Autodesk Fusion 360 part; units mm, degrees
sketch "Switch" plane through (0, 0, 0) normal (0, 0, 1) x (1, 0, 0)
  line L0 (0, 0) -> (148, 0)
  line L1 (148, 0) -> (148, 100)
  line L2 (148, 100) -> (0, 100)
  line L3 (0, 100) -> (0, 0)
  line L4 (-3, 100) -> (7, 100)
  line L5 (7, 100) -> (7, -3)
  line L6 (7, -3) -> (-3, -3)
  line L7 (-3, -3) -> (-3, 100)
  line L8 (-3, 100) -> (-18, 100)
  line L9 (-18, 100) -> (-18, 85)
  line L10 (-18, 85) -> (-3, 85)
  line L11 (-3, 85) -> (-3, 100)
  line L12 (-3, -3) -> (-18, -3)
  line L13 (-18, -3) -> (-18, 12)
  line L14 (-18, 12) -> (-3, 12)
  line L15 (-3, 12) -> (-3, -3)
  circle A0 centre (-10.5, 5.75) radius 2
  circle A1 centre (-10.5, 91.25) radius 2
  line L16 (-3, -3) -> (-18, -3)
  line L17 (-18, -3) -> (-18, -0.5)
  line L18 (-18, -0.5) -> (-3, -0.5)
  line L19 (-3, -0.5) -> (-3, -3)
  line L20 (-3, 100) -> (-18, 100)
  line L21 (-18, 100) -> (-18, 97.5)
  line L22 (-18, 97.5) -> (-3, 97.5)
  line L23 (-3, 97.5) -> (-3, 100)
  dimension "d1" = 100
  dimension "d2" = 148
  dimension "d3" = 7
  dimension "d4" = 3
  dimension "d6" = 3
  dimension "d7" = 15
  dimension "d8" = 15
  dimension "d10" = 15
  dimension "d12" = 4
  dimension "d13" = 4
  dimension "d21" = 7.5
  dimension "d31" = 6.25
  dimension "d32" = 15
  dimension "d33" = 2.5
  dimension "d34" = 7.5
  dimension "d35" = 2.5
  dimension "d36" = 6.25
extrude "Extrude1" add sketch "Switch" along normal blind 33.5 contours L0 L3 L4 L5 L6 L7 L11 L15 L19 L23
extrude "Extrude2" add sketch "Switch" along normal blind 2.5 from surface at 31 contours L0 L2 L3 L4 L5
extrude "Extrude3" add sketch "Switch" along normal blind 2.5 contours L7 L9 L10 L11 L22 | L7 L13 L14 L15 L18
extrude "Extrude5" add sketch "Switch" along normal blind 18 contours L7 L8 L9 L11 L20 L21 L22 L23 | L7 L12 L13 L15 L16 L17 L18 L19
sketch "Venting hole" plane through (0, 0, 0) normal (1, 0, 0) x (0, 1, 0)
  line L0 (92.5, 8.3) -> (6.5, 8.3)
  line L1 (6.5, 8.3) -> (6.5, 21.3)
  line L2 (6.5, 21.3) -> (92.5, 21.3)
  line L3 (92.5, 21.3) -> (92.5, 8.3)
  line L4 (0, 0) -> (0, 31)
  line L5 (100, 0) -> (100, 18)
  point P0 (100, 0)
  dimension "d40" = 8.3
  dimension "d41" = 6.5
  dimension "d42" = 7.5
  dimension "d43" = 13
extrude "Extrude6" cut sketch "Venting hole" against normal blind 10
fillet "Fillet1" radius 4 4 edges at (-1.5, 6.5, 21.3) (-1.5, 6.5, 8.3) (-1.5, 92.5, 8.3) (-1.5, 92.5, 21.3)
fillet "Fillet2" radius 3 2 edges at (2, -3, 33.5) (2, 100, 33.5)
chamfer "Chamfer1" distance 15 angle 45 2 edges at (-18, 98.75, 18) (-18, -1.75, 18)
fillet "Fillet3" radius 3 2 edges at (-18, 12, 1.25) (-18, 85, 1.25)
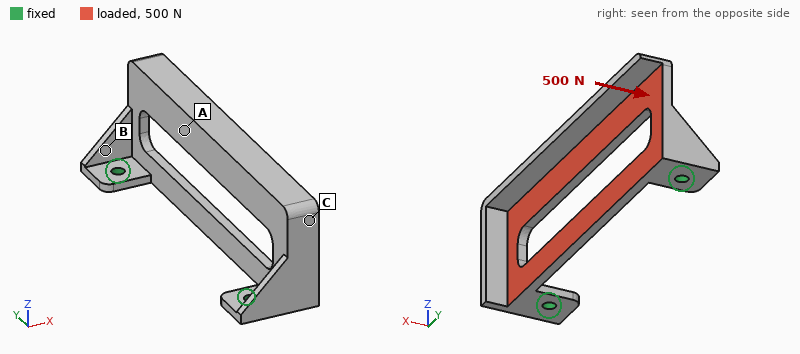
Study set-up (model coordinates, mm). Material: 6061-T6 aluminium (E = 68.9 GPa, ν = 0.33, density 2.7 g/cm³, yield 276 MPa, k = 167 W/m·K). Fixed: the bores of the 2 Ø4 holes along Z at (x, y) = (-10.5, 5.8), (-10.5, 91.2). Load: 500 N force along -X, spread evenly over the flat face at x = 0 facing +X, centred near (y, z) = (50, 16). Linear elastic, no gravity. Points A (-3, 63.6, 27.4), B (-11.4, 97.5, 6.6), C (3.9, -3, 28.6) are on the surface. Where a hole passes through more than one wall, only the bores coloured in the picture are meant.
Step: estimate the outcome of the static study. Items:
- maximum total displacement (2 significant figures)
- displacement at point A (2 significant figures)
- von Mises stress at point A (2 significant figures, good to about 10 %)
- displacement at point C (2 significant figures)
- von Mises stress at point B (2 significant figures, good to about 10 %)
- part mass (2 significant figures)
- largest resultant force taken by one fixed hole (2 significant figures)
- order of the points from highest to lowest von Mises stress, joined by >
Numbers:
0.42 mm
0.35 mm
25 MPa
0.21 mm
53 MPa
30 g
270 N
B > A > C
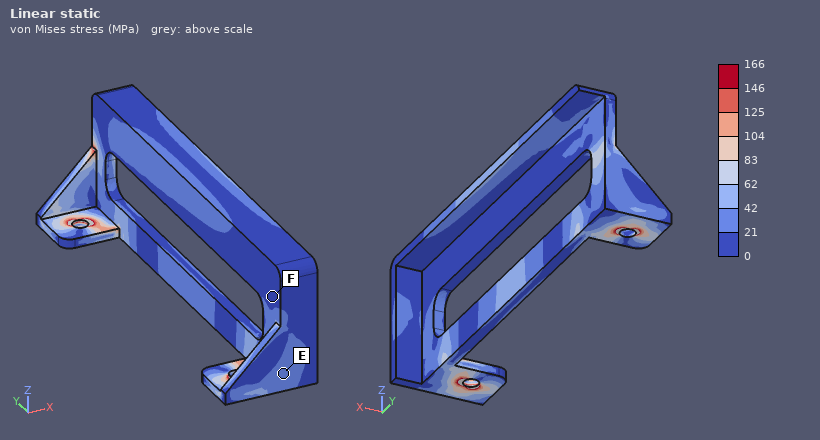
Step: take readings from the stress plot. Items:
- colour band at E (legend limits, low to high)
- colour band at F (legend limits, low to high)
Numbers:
21 to 42 MPa
0 to 21 MPa
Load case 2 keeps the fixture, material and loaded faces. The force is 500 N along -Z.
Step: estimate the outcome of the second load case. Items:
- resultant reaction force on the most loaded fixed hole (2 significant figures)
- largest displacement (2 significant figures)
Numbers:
260 N
0.19 mm
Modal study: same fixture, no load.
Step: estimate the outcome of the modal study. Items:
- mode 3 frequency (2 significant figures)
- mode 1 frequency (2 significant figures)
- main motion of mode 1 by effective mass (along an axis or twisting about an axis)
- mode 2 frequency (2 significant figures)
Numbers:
2400 Hz
1100 Hz
along X
2100 Hz
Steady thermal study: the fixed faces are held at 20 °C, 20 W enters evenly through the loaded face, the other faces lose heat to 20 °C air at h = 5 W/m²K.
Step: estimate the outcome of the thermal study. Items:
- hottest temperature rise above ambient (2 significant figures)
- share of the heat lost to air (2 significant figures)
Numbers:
37 K
4.2 %
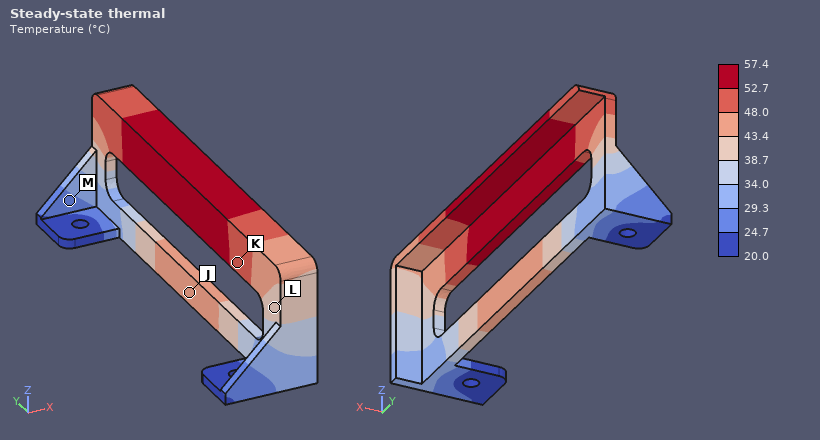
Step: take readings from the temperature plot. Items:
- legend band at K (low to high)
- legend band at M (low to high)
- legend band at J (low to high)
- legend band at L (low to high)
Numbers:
48.0 to 52.7 °C
24.7 to 29.3 °C
43.4 to 48.0 °C
38.7 to 43.4 °C
